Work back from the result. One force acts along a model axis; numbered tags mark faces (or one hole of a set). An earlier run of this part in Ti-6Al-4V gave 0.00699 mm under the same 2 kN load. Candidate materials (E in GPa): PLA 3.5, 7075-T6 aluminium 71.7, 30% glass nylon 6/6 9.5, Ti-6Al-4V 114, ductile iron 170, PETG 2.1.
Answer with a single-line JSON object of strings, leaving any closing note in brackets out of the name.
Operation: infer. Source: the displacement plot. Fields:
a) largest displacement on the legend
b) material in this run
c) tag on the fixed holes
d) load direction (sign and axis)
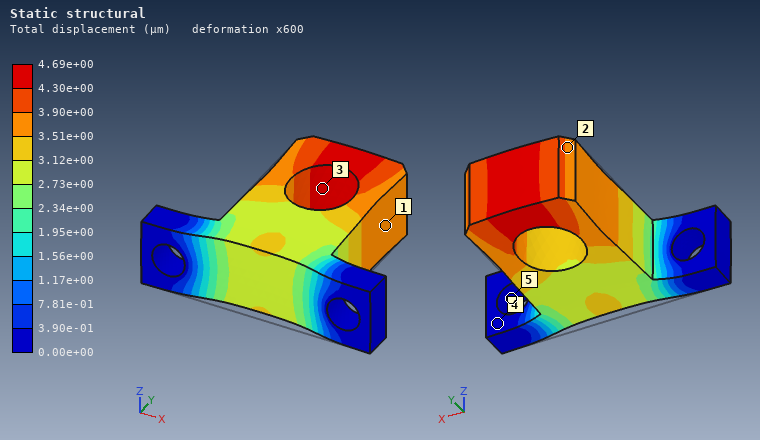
{"largest displacement on the legend": "4.69e+00 µm", "material in this run": "ductile iron", "tag on the fixed holes": "5", "load direction": "+Y"}
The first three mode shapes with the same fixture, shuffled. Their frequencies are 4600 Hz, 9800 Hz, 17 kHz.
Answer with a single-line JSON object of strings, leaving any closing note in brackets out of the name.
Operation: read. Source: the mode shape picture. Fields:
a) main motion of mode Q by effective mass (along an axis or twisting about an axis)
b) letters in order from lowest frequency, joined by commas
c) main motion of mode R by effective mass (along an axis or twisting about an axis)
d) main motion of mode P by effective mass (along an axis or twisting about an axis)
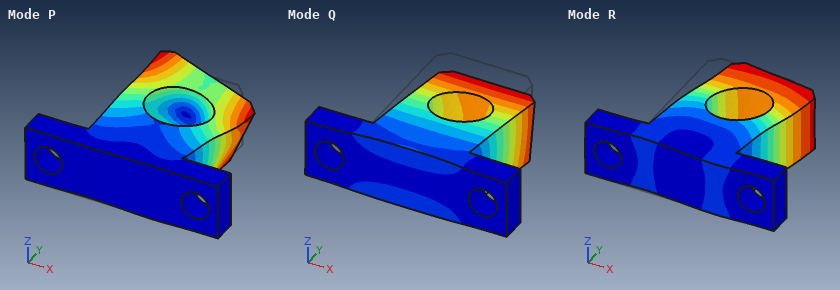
{"main motion of mode Q by effective mass": "along Z", "letters in order from lowest frequency, joined by commas": "Q, R, P", "main motion of mode R by effective mass": "along X", "main motion of mode P by effective mass": "twisting about Y"}
